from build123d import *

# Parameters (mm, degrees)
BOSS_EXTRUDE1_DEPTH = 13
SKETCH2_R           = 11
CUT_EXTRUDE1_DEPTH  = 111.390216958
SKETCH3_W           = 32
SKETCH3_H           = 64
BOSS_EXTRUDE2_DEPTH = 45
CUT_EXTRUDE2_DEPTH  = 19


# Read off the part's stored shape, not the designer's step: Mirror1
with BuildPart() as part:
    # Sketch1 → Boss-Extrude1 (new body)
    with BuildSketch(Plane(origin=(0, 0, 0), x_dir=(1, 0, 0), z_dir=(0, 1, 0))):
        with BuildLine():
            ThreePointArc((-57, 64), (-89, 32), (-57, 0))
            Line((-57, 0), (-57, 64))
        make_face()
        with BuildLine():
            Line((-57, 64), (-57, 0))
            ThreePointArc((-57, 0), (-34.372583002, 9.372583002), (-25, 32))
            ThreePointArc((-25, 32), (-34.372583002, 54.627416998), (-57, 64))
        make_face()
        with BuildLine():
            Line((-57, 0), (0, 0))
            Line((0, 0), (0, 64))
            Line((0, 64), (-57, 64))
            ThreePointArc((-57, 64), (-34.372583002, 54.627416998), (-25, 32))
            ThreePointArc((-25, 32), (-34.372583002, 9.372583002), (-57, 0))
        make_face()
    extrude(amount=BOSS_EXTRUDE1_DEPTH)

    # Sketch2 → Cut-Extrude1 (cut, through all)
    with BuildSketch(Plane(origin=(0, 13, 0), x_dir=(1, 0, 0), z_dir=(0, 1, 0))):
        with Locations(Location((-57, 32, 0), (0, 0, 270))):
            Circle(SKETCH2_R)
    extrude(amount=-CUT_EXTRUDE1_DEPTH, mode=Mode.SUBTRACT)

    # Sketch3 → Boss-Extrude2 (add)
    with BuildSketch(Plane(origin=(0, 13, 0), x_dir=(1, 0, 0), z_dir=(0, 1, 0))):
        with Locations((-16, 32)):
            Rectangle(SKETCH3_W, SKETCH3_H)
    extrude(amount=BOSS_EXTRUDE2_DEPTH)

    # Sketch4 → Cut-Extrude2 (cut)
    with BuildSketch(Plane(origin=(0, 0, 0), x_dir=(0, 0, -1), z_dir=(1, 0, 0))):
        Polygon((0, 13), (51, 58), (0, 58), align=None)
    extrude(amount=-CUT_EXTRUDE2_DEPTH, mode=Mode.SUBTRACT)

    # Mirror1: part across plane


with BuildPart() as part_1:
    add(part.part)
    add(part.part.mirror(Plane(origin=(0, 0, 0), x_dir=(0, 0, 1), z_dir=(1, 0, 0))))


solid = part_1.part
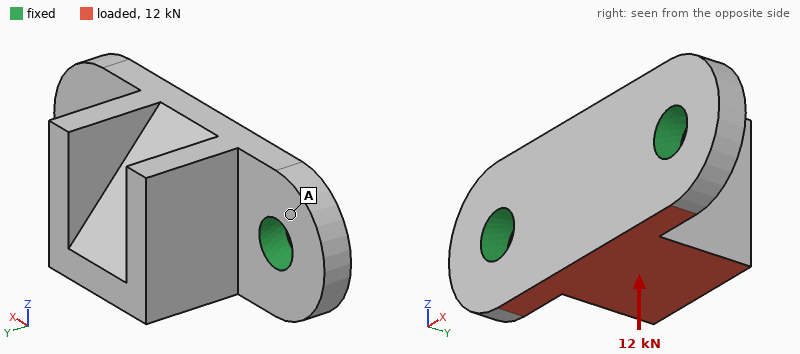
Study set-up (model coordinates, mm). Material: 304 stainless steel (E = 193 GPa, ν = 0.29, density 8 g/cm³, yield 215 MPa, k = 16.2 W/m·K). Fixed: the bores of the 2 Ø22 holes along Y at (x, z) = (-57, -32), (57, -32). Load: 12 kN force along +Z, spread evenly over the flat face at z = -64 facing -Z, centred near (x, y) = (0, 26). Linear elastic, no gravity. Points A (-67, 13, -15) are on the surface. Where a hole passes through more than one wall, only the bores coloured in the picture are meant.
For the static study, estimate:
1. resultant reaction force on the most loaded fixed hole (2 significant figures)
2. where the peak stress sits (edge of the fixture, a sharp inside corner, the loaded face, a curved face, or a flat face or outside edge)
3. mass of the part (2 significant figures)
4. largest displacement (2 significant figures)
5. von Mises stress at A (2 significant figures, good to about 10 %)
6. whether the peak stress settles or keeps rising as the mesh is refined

6.0 kN
edge of the fixture
2.1 kg
38 µm
11 MPa
keeps rising
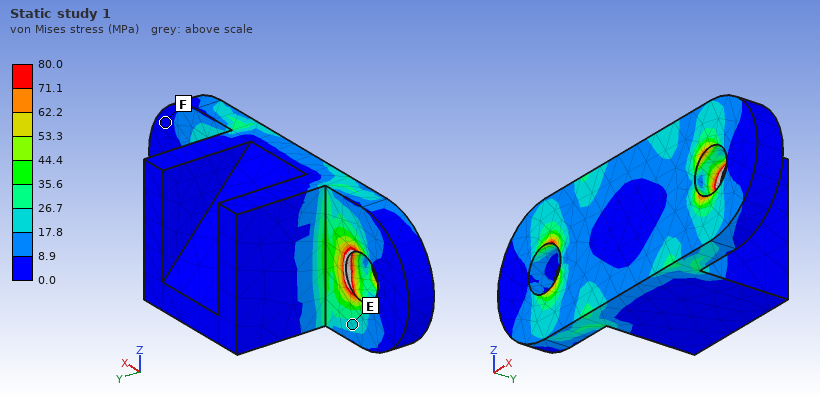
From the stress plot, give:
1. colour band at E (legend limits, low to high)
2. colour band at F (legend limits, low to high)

17.8 to 26.7 MPa
0.0 to 8.9 MPa
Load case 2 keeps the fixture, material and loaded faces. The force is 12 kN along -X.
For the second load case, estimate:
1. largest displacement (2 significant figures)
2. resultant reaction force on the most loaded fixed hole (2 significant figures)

9.4 µm
7.4 kN
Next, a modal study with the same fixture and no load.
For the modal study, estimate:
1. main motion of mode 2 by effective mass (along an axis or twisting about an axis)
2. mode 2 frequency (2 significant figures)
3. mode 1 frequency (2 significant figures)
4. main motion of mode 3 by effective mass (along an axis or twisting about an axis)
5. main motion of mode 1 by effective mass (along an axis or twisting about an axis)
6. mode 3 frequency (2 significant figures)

along Y
4900 Hz
2600 Hz
along X
along Z
5800 Hz
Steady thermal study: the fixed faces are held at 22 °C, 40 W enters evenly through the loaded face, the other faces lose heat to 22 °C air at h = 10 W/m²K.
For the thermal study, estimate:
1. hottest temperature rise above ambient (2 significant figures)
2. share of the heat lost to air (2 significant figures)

55 K
19 %
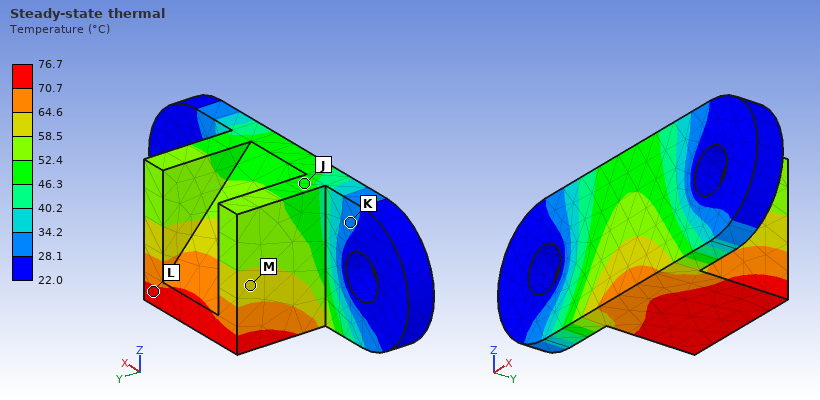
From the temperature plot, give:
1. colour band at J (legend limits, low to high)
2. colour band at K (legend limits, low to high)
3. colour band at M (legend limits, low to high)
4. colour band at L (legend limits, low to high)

46.3 to 52.4 °C
28.1 to 34.2 °C
58.5 to 64.6 °C
70.7 to 76.7 °C
